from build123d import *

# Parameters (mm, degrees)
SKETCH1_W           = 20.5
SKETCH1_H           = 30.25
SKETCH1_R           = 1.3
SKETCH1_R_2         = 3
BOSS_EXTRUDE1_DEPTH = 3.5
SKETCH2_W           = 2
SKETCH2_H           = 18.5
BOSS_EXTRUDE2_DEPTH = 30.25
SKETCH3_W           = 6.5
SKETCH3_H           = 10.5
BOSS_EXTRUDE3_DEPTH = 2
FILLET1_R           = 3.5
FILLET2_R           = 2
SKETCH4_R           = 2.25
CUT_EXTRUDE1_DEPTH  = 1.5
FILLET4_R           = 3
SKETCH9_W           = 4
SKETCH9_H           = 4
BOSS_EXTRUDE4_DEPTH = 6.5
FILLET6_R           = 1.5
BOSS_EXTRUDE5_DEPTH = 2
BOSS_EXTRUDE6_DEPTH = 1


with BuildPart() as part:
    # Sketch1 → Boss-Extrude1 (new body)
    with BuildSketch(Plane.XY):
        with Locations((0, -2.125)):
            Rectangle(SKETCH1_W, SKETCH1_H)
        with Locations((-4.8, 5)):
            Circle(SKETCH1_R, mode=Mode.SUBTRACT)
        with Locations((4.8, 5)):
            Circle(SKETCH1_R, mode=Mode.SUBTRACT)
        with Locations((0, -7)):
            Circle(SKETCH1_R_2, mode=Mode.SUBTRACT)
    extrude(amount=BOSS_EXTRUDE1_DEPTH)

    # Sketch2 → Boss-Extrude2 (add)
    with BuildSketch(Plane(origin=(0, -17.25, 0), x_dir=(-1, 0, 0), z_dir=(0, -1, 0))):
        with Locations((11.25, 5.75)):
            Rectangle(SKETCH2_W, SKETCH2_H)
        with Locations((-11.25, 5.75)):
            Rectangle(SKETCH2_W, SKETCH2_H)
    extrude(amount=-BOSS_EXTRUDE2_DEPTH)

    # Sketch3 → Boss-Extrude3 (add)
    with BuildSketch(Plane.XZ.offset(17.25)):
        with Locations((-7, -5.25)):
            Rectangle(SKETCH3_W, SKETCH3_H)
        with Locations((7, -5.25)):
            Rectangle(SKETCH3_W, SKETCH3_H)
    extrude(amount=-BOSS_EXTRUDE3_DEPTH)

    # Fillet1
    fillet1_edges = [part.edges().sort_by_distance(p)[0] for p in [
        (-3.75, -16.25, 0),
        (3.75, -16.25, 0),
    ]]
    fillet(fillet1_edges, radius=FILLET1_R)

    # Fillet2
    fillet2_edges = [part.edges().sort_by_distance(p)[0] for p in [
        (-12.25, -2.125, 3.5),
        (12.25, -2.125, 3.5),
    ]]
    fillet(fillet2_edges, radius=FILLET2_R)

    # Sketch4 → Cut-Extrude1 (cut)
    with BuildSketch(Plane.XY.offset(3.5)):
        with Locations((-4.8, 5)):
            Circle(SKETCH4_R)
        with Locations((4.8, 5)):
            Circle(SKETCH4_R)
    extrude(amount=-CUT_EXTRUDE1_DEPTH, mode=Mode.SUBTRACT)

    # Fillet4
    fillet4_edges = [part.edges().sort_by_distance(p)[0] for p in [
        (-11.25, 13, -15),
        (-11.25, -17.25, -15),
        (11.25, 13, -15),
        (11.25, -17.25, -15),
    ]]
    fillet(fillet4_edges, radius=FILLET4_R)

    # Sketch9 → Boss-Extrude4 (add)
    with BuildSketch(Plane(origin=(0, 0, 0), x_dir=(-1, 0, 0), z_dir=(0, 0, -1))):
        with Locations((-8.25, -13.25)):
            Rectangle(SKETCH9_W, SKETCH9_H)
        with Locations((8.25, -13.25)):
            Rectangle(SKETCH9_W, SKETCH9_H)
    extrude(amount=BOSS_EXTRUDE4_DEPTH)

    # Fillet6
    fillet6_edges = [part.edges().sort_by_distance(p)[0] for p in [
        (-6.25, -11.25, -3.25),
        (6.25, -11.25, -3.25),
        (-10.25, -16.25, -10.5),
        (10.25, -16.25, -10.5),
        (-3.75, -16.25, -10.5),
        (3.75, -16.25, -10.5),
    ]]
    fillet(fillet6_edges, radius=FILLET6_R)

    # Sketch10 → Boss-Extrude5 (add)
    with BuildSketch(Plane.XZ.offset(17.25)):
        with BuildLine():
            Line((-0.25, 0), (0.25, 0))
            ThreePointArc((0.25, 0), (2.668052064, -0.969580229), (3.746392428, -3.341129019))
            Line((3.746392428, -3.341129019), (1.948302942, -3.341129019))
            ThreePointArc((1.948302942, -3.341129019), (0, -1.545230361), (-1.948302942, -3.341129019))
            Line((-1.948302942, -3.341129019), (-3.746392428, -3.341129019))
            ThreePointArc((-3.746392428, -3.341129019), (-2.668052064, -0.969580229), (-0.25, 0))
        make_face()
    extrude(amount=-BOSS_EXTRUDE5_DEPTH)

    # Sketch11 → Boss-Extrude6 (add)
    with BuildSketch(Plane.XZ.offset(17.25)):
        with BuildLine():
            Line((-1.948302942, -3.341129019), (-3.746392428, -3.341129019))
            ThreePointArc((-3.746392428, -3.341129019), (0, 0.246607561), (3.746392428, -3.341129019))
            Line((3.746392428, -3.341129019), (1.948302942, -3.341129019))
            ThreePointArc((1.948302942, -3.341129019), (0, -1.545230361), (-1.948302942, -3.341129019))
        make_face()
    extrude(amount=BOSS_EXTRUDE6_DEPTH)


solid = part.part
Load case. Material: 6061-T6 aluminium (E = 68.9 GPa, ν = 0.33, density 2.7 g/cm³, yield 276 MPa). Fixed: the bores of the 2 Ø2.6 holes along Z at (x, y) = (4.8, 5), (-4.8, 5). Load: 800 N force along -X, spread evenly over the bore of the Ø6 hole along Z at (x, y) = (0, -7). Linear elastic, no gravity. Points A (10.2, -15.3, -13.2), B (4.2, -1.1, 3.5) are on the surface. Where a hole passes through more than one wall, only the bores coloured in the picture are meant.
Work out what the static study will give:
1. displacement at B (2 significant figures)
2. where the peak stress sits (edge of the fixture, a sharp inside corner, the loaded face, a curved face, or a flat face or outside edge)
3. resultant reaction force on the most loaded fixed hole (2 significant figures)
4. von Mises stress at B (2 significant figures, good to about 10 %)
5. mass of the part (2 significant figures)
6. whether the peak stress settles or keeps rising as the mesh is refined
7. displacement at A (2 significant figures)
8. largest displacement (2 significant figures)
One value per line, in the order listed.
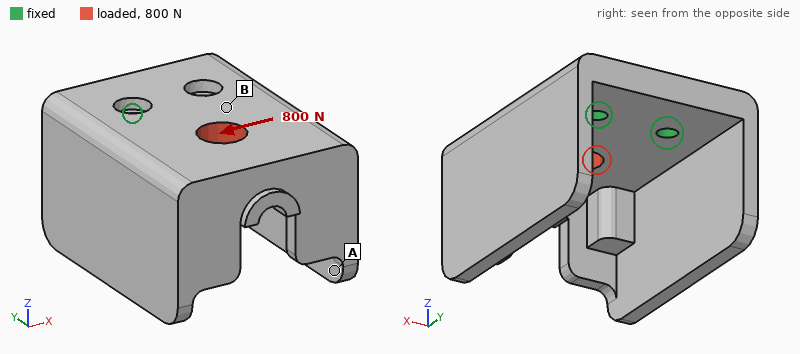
6.5 µm
edge of the fixture
930 N
20 MPa
13 g
keeps rising
23 µm
25 µm
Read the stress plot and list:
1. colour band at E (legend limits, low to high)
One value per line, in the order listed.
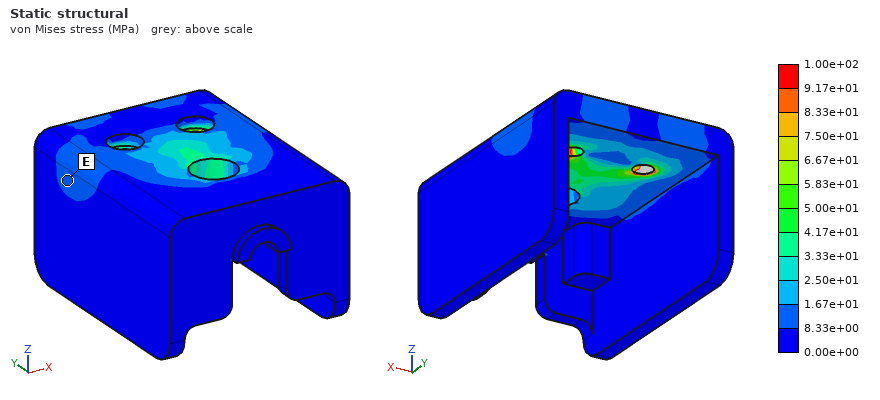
8.33e+00 to 1.67e+01 MPa
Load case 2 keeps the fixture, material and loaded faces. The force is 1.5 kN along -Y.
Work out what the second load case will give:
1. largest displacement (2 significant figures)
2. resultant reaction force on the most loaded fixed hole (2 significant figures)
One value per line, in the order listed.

27 µm
760 N
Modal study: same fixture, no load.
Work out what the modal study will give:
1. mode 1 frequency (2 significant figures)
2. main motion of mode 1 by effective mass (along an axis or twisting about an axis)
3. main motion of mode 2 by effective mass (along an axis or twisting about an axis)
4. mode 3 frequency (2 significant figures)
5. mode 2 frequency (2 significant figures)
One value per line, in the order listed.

3100 Hz
along Z
along X
6600 Hz
4300 Hz
